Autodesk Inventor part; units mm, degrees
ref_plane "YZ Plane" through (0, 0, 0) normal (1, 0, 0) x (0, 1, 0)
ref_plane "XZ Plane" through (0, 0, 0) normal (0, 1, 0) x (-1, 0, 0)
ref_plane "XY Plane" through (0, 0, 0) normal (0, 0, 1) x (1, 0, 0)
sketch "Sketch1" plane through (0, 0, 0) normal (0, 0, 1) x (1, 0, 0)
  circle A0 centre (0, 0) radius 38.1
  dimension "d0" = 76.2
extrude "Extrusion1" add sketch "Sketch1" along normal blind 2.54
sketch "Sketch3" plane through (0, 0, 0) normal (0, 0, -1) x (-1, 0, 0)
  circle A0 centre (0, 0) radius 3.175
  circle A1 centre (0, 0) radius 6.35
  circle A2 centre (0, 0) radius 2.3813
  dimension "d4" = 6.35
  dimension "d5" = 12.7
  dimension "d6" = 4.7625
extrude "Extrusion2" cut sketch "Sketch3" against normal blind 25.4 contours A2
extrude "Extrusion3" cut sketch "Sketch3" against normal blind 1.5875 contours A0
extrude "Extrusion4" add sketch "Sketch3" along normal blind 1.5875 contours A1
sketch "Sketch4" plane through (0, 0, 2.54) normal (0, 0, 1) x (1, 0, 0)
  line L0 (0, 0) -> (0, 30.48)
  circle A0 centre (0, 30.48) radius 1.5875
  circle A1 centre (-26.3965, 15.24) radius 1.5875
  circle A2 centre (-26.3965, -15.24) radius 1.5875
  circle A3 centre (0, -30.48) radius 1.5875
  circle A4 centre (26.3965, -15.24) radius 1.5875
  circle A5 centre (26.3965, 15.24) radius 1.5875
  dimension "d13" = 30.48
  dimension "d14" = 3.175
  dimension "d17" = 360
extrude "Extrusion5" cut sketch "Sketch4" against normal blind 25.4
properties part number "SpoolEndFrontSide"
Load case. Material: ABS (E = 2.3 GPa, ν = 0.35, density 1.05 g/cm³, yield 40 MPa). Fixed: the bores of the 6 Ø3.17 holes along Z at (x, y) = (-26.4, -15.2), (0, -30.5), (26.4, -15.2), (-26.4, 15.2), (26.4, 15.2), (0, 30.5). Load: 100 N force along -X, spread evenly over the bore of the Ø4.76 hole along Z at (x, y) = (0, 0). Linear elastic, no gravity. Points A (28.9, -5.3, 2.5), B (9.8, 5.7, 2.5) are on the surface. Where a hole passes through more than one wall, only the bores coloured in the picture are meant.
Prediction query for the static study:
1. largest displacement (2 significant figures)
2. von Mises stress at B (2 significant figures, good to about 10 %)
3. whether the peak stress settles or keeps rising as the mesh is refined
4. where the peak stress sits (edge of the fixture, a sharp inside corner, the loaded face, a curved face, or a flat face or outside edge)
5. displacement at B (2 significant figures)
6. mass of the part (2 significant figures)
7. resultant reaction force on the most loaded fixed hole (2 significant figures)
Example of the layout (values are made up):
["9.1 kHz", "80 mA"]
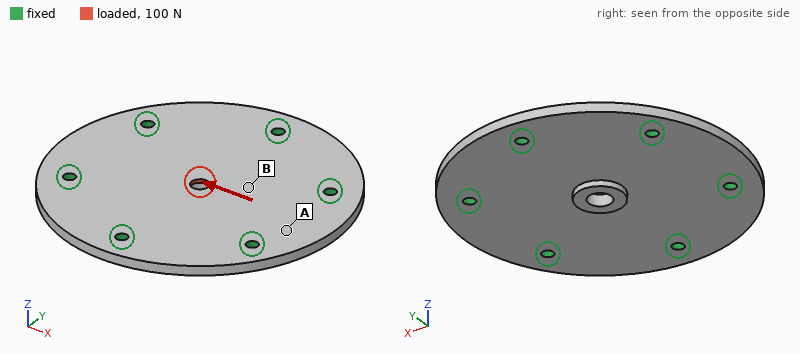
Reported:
["21 µm", "1.3 MPa", "keeps rising", "a sharp inside corner", "11 µm", "12 g", "22 N"]
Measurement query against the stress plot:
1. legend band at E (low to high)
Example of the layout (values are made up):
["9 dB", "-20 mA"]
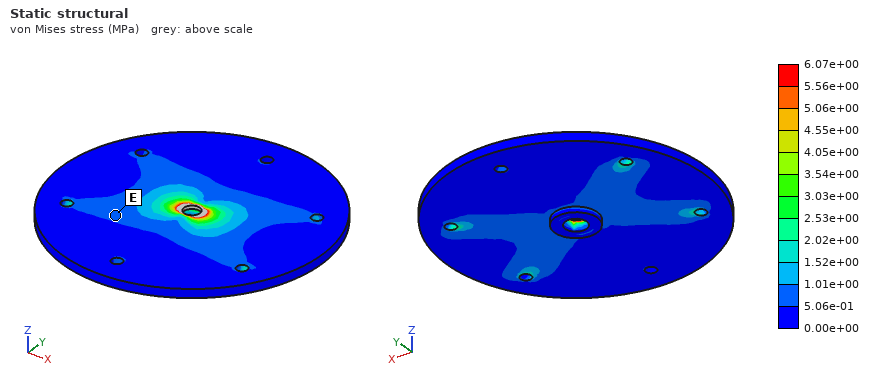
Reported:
["5.06e-01 to 1.01e+00 MPa"]
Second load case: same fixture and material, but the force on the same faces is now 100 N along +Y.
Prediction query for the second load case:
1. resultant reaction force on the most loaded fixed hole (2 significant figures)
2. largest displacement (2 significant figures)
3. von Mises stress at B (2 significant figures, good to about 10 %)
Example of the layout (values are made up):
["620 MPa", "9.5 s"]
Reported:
["25 N", "20 µm", "0.90 MPa"]
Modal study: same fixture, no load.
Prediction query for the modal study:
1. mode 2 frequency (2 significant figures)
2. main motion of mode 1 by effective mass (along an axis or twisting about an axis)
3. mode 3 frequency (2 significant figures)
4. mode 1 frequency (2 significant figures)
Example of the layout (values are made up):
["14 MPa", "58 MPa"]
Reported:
["3100 Hz", "along Z", "3200 Hz", "1700 Hz"]
